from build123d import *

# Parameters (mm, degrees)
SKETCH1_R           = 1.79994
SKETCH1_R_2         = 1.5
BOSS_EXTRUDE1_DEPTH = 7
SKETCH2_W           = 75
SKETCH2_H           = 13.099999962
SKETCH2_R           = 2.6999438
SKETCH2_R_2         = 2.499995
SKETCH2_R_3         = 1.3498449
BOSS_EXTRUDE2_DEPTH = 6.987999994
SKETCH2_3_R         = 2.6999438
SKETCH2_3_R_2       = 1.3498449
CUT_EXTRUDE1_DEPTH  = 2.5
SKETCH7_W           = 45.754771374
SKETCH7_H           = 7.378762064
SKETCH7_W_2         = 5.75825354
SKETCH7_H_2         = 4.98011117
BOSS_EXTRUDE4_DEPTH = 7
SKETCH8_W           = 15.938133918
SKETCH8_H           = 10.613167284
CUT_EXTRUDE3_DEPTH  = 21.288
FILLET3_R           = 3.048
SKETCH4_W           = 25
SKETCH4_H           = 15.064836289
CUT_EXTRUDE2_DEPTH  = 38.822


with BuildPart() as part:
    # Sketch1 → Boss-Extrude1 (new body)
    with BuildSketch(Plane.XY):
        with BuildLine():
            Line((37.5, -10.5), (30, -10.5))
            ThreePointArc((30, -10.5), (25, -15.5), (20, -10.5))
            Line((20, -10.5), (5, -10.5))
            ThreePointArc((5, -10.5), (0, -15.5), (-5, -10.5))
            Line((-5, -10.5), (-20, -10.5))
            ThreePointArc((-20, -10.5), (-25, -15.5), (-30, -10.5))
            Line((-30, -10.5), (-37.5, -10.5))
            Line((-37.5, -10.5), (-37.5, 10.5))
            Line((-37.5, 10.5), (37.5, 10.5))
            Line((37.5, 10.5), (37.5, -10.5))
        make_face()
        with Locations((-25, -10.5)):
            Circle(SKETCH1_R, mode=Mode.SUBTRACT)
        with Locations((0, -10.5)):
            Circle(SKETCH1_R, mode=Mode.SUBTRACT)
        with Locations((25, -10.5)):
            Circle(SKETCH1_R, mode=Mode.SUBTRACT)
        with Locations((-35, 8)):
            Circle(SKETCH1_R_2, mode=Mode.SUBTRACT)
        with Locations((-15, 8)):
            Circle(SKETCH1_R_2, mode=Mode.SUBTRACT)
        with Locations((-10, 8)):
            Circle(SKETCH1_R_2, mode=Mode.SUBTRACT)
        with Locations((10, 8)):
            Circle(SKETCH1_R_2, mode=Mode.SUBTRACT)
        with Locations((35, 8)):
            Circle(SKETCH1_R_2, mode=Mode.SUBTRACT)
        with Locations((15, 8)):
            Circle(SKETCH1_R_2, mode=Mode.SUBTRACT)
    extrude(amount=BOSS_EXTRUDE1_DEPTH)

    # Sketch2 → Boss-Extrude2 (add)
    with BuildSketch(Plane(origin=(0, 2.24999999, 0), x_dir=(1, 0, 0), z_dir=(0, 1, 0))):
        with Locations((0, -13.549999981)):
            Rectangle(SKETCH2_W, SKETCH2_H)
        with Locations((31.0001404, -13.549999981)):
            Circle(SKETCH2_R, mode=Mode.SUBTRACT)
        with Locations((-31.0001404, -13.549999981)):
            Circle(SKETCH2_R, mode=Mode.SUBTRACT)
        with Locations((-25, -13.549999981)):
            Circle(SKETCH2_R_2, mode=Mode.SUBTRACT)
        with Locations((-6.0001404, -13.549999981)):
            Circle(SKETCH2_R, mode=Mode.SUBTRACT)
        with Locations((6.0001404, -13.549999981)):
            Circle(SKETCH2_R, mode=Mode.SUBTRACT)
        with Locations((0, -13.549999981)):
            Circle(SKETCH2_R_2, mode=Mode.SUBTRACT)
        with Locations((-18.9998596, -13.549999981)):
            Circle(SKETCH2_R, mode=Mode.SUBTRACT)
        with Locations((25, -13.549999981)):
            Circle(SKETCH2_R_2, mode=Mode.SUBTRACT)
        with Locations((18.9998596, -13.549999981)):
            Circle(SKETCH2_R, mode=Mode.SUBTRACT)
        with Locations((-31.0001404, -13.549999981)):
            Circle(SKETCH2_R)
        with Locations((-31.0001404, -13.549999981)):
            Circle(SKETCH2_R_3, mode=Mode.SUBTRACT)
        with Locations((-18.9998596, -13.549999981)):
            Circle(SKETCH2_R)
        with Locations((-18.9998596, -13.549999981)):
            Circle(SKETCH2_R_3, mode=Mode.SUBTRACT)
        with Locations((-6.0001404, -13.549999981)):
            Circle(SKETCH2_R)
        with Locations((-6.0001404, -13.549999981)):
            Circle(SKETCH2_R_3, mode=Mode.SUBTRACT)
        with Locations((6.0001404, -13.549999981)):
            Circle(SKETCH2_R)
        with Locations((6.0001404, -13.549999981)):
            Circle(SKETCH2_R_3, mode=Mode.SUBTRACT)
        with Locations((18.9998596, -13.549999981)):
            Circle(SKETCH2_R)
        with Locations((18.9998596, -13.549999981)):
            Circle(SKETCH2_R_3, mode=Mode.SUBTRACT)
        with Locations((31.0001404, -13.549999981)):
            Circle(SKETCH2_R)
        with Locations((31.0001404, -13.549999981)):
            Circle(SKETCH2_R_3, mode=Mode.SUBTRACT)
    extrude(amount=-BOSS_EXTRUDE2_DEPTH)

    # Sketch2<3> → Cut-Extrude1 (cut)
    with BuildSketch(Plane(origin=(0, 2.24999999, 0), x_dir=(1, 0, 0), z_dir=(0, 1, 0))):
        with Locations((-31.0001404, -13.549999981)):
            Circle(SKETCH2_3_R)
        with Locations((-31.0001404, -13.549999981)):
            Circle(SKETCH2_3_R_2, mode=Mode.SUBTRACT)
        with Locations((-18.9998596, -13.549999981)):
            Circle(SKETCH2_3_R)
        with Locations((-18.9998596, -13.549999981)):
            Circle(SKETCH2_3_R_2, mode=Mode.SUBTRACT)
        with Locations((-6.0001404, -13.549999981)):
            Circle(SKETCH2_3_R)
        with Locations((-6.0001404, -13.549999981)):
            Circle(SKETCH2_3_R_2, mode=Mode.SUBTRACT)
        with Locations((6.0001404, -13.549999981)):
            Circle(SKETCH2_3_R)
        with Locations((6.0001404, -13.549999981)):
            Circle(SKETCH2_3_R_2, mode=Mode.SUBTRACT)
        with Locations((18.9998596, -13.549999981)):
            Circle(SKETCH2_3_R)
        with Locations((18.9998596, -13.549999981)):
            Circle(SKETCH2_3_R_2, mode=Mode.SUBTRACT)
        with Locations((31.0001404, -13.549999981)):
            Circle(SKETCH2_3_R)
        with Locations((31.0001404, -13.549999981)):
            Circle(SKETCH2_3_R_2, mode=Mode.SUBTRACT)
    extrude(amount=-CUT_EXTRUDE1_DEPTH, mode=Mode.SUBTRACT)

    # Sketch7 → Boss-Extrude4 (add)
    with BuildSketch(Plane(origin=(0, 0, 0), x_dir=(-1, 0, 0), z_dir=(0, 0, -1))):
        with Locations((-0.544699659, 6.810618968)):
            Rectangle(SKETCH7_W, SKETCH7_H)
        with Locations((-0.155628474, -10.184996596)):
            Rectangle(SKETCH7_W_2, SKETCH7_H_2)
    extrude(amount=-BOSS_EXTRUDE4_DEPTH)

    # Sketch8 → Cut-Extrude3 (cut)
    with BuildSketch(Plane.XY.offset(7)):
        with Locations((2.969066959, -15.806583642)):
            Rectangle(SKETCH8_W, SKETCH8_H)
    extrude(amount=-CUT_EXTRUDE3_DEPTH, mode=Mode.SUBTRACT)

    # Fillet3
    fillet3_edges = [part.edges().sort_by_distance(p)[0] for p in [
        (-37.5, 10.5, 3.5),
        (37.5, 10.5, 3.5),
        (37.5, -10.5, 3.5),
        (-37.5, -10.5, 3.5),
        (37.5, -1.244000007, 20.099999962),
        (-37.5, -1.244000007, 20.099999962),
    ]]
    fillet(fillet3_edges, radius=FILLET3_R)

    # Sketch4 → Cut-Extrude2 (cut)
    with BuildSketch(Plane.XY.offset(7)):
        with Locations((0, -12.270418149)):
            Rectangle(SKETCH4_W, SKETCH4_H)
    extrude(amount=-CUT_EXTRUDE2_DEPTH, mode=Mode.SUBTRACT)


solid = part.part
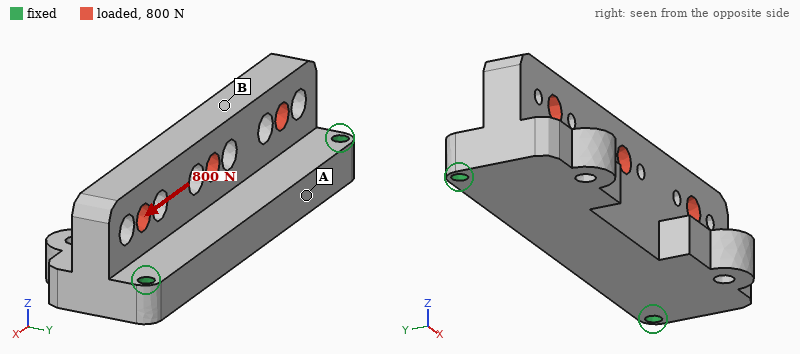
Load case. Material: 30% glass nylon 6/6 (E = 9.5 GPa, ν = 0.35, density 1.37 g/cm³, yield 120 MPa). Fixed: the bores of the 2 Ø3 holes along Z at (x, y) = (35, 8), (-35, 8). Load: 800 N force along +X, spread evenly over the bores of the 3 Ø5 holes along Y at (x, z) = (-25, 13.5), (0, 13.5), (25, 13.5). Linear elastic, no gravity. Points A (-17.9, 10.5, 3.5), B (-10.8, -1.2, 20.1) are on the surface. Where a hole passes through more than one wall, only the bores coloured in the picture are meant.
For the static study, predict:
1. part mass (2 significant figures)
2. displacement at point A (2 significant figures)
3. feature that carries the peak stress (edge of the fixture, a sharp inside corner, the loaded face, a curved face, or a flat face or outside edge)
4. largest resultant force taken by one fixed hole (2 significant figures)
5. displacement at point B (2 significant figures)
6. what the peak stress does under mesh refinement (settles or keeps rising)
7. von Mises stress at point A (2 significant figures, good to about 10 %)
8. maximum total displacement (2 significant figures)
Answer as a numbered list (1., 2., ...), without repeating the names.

1. 22 g
2. 10 µm
3. edge of the fixture
4. 430 N
5. 25 µm
6. keeps rising
7. 4.3 MPa
8. 35 µm
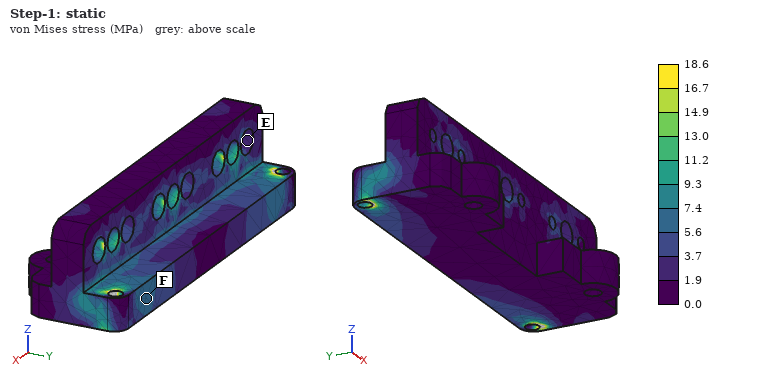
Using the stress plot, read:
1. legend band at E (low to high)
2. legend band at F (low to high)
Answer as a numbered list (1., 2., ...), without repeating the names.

1. 1.9 to 3.7 MPa
2. 5.6 to 7.4 MPa
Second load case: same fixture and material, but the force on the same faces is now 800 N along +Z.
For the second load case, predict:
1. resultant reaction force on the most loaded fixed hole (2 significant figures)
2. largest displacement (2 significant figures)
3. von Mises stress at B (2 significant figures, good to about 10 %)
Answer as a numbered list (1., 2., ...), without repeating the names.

1. 400 N
2. 0.21 mm
3. 7.6 MPa
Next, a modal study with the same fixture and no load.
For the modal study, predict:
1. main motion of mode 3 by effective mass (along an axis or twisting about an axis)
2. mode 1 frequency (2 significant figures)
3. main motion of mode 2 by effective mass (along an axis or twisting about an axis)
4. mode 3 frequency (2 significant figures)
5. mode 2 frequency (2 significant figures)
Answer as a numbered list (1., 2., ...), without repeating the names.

1. along Z
2. 2400 Hz
3. along Y
4. 4700 Hz
5. 4500 Hz
